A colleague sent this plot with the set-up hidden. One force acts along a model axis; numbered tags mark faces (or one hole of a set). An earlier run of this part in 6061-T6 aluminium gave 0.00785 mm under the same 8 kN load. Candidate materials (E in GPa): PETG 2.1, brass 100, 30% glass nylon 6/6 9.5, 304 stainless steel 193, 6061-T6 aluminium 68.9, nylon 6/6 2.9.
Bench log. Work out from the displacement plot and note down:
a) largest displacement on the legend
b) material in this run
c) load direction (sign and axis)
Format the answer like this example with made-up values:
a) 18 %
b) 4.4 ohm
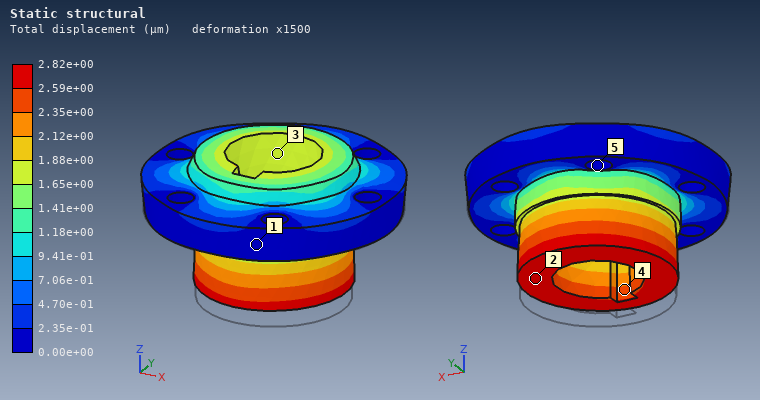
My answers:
a) 2.82e+00 µm
b) 304 stainless steel
c) +Z
